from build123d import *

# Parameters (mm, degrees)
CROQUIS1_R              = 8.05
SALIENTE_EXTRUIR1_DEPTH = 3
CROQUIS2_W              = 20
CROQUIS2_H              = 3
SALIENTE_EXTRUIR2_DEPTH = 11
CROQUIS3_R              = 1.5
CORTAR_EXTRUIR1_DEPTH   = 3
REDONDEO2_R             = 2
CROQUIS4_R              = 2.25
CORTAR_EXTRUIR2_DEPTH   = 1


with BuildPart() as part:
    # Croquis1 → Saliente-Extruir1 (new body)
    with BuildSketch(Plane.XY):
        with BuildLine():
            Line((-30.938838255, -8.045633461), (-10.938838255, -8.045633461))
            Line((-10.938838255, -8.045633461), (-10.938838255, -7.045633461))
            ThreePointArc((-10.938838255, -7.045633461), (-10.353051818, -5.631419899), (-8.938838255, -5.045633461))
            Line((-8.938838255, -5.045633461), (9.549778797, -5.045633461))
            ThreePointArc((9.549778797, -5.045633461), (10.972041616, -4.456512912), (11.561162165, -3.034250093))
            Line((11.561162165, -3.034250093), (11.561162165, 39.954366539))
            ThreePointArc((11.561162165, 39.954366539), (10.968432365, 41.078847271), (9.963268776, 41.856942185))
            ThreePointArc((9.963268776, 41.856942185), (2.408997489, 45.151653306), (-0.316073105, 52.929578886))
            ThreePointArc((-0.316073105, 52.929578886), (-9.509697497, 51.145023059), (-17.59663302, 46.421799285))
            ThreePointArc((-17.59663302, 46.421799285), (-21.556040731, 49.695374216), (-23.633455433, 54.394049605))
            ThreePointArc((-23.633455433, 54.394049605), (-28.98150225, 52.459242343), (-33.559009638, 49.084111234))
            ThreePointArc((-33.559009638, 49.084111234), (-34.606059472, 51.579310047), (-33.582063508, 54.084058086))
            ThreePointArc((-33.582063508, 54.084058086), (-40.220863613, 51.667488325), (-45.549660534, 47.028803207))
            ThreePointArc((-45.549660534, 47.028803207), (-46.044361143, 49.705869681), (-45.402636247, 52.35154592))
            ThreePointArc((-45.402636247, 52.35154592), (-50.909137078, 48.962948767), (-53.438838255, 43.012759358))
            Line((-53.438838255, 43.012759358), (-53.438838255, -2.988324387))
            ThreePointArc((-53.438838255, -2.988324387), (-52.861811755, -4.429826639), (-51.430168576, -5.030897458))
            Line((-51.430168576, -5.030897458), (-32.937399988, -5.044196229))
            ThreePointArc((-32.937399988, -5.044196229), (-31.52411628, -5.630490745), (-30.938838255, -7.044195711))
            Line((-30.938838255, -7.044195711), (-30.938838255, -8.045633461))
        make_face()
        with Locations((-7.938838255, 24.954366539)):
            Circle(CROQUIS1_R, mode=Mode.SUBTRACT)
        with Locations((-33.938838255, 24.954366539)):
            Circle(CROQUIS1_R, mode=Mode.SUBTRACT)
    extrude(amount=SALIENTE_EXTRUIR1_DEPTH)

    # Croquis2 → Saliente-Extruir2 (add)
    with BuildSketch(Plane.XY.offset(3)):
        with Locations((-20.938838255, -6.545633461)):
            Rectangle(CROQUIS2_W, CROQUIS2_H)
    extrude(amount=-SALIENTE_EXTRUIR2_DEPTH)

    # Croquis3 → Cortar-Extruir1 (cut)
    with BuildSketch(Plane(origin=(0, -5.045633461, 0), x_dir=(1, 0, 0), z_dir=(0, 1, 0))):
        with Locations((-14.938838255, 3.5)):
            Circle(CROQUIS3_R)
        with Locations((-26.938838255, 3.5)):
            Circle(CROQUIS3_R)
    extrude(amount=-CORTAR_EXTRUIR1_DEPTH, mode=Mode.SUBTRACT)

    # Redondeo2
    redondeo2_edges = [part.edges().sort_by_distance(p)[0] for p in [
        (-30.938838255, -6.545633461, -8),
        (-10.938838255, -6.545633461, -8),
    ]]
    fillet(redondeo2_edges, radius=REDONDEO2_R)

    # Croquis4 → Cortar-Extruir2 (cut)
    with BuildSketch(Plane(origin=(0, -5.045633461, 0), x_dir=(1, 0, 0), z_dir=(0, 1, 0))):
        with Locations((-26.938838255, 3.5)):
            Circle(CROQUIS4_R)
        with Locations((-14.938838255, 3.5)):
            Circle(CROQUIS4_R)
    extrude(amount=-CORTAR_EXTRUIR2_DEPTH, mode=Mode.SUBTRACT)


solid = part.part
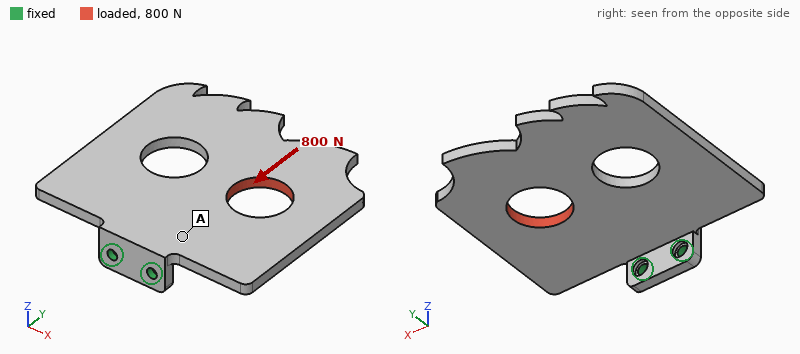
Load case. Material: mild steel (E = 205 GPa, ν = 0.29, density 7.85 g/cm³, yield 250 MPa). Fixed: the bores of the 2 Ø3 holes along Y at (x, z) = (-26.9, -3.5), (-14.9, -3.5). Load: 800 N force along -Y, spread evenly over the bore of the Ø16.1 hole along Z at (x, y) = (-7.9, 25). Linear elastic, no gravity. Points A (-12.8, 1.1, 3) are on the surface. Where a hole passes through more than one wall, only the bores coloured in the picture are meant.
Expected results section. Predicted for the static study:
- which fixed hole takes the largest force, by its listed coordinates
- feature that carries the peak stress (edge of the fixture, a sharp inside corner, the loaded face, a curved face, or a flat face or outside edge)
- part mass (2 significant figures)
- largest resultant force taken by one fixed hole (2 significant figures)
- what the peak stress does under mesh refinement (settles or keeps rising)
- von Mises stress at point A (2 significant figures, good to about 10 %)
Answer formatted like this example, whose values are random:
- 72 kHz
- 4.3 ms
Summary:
- (-14.9, -3.5)
- edge of the fixture
- 79 g
- 1.2 kN
- keeps rising
- 20 MPa
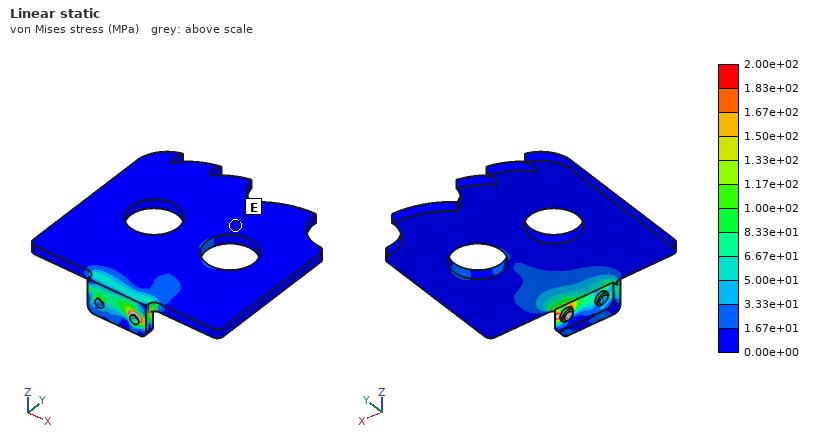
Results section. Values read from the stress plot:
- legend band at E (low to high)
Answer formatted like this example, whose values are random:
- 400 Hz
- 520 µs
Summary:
- 0.00e+00 to 1.67e+01 MPa
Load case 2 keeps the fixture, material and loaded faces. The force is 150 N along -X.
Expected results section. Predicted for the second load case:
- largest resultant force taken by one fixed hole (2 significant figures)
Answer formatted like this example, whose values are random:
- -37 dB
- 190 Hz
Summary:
- 370 N
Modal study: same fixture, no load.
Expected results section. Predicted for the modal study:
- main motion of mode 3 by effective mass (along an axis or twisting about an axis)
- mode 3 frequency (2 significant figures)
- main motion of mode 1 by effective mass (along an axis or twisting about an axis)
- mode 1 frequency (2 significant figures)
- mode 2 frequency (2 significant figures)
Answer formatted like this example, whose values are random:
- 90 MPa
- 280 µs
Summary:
- along X
- 1600 Hz
- along Z
- 460 Hz
- 1000 Hz
